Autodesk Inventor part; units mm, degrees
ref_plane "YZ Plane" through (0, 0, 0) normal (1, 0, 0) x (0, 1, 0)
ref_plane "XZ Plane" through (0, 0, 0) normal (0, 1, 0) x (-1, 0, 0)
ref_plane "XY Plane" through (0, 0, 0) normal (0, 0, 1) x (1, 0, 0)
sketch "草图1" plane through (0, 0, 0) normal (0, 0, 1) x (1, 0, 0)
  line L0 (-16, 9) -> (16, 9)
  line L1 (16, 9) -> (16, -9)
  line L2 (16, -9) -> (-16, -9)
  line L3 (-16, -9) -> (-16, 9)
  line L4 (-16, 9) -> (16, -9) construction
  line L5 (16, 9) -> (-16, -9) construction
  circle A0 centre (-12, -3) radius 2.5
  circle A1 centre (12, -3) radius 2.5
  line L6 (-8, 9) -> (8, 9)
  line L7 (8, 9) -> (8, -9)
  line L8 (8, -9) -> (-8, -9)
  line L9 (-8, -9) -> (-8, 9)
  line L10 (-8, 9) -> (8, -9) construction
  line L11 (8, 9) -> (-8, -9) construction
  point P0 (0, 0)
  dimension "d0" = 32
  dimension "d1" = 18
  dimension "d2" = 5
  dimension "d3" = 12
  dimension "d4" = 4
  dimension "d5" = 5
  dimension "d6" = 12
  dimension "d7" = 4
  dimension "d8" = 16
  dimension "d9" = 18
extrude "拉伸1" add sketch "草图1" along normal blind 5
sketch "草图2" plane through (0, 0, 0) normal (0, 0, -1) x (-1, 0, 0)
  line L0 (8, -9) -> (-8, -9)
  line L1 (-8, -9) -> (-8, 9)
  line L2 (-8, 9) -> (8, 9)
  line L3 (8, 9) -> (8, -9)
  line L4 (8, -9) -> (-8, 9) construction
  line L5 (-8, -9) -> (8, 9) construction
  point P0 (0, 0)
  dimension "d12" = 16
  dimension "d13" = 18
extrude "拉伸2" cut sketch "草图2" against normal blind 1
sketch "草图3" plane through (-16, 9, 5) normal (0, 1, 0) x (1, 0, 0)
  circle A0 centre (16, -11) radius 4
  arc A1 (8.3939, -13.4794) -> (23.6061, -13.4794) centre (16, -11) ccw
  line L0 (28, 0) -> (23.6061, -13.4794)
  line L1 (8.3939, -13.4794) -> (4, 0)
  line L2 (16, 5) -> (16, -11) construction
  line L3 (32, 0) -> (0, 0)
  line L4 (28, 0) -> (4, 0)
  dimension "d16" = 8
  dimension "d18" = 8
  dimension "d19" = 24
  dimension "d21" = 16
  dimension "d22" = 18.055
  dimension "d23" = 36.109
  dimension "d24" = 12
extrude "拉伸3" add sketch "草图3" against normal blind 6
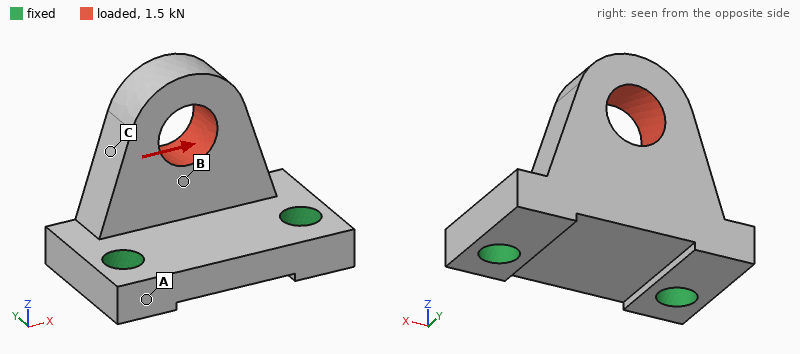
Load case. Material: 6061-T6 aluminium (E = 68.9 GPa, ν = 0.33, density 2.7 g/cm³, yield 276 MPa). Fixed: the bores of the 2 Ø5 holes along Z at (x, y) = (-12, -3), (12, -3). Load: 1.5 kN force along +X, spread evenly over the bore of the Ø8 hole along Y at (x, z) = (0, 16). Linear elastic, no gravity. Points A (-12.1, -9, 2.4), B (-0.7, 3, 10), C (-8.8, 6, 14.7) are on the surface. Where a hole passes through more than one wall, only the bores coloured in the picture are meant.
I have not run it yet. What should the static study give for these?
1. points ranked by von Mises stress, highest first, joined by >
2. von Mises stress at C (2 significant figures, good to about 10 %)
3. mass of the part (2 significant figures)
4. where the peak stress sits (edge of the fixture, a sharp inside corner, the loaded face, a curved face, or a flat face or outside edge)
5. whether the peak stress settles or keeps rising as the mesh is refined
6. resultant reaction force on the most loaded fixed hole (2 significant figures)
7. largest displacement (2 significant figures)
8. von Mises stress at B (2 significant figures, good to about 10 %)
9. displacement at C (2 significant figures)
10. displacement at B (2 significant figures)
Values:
B > C > A
34 MPa
11 g
edge of the fixture
keeps rising
1.2 kN
44 µm
58 MPa
28 µm
15 µm
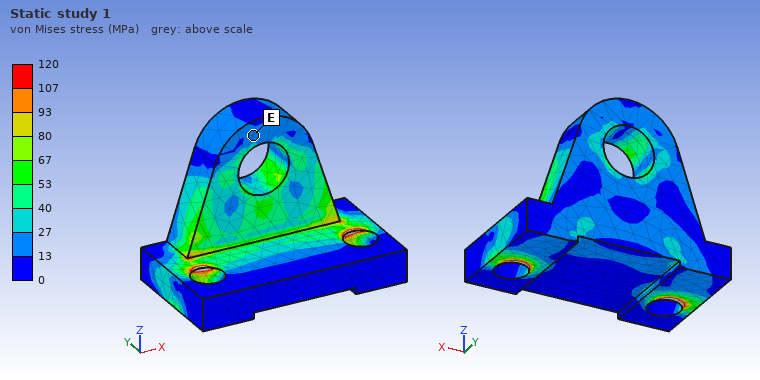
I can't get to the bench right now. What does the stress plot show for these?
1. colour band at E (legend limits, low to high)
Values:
13 to 27 MPa
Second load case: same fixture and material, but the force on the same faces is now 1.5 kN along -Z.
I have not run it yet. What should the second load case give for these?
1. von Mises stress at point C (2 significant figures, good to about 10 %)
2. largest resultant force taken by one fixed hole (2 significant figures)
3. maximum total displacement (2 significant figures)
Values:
17 MPa
760 N
72 µm
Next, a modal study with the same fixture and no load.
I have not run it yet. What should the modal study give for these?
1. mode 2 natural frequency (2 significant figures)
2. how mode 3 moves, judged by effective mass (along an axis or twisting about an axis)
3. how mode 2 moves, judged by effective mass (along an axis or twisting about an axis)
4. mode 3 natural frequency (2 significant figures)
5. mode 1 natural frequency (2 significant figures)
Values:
18 kHz
along Z
along X
22 kHz
8000 Hz
